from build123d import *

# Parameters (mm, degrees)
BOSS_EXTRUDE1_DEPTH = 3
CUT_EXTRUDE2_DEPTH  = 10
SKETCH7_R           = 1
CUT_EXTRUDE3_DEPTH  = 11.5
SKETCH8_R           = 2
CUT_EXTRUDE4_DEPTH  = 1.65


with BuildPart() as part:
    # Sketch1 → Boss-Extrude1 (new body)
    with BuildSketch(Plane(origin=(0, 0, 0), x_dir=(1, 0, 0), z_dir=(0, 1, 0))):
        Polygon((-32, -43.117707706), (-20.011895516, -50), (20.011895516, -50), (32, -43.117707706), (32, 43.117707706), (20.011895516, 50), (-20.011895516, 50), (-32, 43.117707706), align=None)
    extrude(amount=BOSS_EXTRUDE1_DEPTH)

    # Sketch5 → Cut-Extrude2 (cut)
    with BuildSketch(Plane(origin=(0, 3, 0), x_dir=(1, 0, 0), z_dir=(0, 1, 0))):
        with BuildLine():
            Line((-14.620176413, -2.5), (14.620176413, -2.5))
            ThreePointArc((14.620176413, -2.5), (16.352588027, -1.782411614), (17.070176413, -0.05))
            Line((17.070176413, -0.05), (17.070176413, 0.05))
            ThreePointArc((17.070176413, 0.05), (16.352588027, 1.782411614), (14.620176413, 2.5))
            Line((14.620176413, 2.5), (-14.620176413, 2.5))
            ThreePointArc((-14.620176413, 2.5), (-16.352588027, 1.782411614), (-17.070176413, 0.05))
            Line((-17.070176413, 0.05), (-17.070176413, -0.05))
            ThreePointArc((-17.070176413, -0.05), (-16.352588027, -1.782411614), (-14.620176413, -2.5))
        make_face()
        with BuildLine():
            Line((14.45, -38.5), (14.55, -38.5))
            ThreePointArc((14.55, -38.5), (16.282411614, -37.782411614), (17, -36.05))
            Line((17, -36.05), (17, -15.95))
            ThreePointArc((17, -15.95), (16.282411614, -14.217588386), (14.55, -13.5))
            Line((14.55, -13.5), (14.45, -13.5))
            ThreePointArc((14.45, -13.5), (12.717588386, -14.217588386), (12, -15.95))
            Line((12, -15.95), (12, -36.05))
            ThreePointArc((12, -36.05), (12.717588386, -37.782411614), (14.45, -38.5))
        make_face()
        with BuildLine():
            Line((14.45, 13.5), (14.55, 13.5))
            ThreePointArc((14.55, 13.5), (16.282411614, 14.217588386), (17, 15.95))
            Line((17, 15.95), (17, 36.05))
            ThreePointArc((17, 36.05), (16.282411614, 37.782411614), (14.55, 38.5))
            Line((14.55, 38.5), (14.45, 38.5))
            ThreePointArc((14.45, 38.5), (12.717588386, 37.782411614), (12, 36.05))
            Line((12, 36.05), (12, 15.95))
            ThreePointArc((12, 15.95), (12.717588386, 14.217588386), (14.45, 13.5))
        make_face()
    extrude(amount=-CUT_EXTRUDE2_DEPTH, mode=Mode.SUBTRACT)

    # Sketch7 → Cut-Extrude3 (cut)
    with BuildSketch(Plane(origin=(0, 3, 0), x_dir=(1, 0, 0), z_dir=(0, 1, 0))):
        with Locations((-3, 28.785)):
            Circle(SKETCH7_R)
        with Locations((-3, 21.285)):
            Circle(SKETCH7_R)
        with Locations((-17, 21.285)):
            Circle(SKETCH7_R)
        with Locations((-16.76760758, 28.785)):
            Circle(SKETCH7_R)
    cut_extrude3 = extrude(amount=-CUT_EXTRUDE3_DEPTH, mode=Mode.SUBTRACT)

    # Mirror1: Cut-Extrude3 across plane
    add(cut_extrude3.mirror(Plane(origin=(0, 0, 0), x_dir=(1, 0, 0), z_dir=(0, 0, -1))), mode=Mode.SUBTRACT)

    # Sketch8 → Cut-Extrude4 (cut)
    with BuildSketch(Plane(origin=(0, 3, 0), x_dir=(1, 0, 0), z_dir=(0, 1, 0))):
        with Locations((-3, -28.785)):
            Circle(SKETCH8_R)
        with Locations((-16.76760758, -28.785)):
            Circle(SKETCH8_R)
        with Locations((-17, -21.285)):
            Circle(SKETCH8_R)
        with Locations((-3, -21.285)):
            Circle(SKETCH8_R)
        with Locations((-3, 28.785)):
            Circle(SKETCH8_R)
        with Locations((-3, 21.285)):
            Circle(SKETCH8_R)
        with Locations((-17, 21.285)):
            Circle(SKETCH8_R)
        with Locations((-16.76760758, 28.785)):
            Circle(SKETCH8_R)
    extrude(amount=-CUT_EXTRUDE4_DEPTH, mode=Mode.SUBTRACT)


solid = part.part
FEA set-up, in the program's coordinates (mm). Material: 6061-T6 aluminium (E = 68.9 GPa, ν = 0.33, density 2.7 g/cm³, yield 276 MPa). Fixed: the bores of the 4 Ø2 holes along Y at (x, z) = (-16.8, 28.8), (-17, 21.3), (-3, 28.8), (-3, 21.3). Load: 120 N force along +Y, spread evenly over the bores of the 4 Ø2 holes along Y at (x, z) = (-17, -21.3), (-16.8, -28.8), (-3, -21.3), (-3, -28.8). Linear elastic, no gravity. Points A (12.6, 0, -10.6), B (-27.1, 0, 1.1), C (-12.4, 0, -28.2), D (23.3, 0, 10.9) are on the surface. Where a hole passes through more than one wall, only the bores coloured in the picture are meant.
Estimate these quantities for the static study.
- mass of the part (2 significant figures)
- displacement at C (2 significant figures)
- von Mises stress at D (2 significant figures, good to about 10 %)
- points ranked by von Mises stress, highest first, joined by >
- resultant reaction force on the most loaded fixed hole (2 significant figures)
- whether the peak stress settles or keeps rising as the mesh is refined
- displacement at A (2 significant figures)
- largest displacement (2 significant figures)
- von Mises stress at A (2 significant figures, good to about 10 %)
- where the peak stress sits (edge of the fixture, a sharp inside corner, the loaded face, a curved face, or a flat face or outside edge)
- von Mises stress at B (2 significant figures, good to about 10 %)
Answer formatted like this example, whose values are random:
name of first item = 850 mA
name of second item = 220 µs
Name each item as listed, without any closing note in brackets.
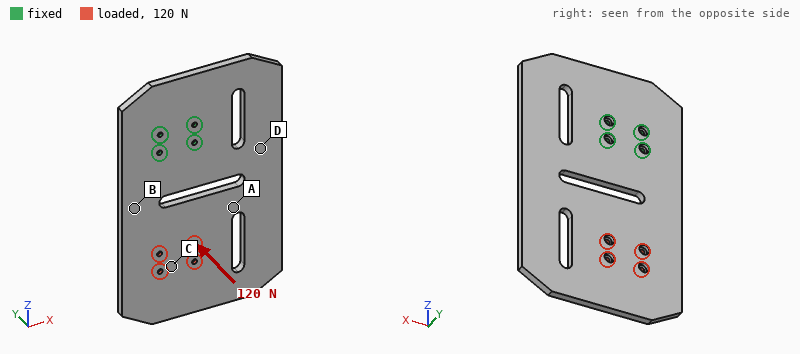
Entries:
mass of the part = 47 g
displacement at C = 0.85 mm
von Mises stress at D = 43 MPa
points ranked by von Mises stress, highest first, joined by > = B > D > A > C
resultant reaction force on the most loaded fixed hole = 400 N
whether the peak stress settles or keeps rising as the mesh is refined = keeps rising
displacement at A = 0.43 mm
largest displacement = 1.4 mm
von Mises stress at A = 26 MPa
where the peak stress sits = edge of the fixture
von Mises stress at B = 67 MPa
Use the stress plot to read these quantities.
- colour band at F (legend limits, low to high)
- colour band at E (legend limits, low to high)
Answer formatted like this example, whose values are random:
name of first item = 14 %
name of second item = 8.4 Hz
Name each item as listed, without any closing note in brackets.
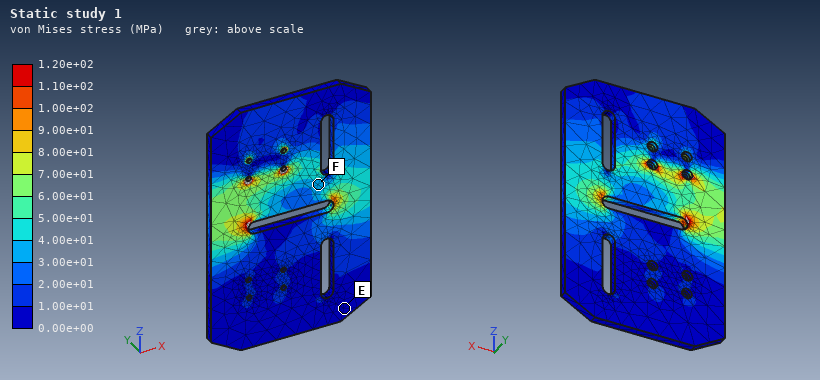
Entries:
colour band at F = 3.00e+01 to 4.00e+01 MPa
colour band at E = 0.00e+00 to 1.00e+01 MPa
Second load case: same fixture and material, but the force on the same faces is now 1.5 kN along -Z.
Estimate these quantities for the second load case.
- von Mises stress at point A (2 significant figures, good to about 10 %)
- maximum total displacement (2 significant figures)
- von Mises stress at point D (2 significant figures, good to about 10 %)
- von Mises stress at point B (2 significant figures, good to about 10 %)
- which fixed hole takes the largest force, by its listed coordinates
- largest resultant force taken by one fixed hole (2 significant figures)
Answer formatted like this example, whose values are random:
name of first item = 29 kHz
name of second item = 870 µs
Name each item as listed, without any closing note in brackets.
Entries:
von Mises stress at point A = 32 MPa
maximum total displacement = 0.45 mm
von Mises stress at point D = 21 MPa
von Mises stress at point B = 41 MPa
which fixed hole takes the largest force, by its listed coordinates = (-17, 21.3)
largest resultant force taken by one fixed hole = 510 N
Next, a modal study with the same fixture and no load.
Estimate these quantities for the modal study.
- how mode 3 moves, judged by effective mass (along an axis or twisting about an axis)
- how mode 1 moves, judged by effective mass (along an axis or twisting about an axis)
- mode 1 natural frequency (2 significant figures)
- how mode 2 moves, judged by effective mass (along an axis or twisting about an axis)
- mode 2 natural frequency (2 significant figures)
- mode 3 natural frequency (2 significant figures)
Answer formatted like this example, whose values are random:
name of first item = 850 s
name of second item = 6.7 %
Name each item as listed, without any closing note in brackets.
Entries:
how mode 3 moves, judged by effective mass = along Y
how mode 1 moves, judged by effective mass = along Y
mode 1 natural frequency = 370 Hz
how mode 2 moves, judged by effective mass = twisting about Z
mode 2 natural frequency = 930 Hz
mode 3 natural frequency = 1800 Hz
